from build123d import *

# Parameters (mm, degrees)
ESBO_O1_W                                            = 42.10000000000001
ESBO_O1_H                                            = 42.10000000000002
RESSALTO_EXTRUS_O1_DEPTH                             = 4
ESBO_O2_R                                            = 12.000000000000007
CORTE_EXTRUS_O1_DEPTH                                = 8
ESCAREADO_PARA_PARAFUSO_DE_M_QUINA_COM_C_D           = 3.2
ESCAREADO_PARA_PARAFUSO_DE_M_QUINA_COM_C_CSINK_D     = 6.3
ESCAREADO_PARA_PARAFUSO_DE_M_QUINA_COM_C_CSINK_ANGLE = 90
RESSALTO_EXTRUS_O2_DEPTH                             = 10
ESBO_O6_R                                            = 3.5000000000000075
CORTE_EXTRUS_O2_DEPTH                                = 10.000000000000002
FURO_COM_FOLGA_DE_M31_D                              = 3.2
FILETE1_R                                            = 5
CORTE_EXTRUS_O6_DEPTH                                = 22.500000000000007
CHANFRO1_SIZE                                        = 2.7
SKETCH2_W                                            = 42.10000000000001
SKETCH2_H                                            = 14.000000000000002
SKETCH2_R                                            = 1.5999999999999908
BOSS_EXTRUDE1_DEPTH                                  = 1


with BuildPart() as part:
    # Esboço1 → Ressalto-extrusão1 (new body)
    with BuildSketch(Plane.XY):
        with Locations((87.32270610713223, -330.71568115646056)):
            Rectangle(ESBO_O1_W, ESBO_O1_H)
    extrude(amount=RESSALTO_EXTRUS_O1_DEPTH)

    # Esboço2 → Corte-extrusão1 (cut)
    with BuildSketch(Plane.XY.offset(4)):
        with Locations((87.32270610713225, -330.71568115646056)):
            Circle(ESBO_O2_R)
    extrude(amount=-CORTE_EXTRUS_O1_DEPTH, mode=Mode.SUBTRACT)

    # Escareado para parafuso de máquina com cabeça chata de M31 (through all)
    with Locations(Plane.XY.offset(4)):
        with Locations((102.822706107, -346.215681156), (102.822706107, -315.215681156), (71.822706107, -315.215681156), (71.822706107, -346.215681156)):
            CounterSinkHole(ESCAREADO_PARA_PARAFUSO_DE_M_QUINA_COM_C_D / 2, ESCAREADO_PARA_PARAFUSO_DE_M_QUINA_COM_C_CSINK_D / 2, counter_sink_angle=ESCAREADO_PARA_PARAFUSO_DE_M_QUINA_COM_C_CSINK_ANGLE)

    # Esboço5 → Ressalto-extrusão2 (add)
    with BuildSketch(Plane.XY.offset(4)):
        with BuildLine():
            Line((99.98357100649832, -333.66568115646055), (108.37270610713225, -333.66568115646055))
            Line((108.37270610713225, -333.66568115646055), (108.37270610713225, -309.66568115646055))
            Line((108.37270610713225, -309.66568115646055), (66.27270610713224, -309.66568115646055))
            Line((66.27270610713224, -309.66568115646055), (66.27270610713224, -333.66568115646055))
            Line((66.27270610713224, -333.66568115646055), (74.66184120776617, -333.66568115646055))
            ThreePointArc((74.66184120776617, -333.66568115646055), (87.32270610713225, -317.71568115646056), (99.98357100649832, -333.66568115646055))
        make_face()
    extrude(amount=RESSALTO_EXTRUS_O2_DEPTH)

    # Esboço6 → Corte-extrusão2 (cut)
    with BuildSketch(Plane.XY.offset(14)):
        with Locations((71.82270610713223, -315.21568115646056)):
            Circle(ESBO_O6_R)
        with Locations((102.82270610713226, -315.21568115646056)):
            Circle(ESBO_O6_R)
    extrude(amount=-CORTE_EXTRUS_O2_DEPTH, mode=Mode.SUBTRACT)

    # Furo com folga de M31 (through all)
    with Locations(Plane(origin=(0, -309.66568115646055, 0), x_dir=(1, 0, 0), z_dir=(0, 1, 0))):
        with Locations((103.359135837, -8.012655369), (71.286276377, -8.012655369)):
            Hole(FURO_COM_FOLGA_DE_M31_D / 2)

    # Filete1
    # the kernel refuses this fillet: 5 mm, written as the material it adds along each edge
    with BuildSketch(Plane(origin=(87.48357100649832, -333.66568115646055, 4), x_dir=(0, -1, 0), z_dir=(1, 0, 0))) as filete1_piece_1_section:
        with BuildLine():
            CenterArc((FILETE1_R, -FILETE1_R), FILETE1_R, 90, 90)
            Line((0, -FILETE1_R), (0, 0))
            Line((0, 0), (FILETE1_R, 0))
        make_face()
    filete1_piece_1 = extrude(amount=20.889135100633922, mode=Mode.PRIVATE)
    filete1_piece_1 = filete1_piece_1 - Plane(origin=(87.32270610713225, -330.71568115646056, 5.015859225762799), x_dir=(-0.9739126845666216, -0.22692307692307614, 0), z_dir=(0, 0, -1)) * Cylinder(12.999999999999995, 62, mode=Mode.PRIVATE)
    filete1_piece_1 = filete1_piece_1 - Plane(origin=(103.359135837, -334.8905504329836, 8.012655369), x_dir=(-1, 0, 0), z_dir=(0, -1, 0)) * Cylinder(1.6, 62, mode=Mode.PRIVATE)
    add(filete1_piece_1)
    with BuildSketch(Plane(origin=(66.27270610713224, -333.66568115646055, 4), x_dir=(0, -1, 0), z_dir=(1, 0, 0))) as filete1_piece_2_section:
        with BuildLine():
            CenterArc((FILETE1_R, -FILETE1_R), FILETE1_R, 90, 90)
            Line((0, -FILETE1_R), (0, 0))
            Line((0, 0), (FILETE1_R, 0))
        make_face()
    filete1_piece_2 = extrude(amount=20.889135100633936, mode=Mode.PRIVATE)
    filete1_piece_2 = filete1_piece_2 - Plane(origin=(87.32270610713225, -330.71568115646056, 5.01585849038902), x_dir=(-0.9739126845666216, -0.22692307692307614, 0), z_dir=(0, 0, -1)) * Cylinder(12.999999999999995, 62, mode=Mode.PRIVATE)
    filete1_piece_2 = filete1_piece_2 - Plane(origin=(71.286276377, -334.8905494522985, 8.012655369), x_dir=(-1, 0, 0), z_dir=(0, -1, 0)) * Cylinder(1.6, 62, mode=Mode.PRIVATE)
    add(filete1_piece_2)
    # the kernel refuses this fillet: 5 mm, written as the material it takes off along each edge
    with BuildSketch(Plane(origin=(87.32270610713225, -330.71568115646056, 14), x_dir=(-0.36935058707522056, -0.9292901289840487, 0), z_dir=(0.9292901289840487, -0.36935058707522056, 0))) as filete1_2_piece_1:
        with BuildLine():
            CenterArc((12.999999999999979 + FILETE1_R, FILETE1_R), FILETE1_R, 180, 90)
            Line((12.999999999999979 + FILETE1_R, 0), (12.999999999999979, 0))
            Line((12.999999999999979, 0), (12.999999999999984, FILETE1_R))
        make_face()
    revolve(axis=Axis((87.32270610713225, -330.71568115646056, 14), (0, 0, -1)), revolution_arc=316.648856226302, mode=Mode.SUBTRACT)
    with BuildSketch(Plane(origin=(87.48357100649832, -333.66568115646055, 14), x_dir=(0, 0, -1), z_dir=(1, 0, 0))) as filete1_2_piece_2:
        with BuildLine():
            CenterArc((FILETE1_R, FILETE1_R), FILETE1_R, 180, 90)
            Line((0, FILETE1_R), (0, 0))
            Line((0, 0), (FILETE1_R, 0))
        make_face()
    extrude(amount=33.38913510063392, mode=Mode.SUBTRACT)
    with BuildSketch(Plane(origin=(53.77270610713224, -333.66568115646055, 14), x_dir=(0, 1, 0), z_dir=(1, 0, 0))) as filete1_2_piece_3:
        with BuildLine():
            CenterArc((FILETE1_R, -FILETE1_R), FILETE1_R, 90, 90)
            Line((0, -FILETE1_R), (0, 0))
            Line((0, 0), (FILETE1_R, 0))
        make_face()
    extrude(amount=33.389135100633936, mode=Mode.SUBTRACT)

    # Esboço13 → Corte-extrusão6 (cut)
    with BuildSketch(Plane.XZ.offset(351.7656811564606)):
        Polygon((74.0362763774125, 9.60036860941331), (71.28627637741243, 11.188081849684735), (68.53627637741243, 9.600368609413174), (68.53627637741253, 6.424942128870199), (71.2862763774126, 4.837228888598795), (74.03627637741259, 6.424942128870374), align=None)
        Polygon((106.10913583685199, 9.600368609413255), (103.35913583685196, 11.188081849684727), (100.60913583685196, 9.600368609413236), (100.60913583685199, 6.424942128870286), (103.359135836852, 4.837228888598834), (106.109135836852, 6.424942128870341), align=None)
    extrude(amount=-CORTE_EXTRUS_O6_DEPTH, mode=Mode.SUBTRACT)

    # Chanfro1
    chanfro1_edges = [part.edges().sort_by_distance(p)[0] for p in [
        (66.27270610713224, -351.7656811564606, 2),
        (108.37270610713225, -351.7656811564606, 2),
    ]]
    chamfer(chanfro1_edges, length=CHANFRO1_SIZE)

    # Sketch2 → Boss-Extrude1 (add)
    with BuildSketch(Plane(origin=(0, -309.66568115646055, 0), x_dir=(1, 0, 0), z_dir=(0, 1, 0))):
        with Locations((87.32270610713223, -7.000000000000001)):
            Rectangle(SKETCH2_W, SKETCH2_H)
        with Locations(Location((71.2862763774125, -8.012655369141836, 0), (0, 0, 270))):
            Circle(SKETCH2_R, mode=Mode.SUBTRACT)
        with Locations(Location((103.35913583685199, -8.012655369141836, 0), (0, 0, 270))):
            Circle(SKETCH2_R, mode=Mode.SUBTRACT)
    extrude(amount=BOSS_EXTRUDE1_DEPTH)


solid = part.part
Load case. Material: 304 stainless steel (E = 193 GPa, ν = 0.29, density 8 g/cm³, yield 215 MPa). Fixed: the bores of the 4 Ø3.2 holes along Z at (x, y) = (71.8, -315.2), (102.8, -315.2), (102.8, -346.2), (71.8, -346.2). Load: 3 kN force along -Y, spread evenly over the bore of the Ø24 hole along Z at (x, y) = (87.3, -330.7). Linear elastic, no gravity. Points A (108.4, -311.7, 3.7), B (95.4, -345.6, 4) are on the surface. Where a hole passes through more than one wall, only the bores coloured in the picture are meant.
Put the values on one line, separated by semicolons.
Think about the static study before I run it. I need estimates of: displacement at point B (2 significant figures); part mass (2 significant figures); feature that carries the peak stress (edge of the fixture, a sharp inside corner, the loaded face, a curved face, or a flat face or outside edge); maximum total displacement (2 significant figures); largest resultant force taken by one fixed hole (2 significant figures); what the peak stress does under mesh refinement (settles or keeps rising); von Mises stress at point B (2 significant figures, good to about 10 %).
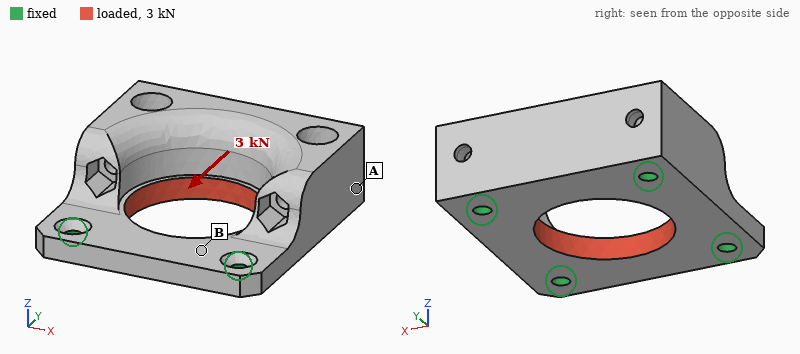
1.8 µm; 87 g; edge of the fixture; 3.1 µm; 780 N; keeps rising; 16 MPa
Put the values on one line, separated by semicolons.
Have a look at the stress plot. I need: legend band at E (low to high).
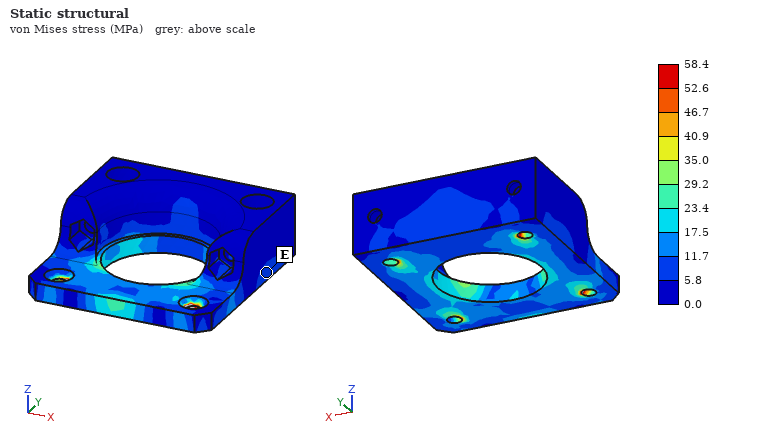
5.8 to 11.7 MPa
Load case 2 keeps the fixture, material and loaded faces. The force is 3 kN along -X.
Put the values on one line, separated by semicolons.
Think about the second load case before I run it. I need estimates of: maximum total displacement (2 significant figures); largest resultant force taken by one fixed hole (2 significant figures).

2.3 µm; 800 N
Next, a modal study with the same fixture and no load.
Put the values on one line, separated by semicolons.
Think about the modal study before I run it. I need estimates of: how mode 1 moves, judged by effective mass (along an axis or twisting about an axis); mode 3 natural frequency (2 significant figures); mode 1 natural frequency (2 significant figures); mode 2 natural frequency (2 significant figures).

along Y; 18 kHz; 13 kHz; 18 kHz
